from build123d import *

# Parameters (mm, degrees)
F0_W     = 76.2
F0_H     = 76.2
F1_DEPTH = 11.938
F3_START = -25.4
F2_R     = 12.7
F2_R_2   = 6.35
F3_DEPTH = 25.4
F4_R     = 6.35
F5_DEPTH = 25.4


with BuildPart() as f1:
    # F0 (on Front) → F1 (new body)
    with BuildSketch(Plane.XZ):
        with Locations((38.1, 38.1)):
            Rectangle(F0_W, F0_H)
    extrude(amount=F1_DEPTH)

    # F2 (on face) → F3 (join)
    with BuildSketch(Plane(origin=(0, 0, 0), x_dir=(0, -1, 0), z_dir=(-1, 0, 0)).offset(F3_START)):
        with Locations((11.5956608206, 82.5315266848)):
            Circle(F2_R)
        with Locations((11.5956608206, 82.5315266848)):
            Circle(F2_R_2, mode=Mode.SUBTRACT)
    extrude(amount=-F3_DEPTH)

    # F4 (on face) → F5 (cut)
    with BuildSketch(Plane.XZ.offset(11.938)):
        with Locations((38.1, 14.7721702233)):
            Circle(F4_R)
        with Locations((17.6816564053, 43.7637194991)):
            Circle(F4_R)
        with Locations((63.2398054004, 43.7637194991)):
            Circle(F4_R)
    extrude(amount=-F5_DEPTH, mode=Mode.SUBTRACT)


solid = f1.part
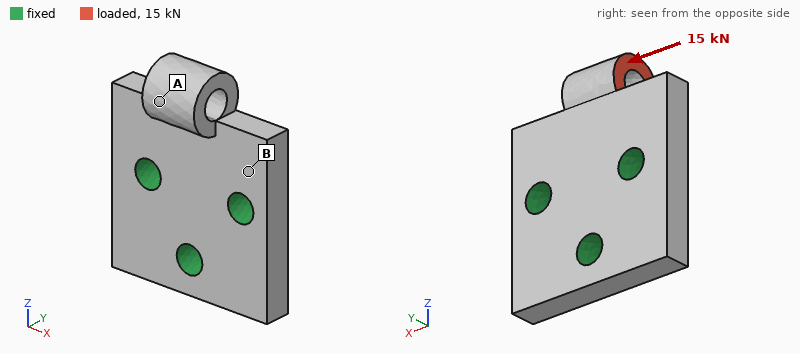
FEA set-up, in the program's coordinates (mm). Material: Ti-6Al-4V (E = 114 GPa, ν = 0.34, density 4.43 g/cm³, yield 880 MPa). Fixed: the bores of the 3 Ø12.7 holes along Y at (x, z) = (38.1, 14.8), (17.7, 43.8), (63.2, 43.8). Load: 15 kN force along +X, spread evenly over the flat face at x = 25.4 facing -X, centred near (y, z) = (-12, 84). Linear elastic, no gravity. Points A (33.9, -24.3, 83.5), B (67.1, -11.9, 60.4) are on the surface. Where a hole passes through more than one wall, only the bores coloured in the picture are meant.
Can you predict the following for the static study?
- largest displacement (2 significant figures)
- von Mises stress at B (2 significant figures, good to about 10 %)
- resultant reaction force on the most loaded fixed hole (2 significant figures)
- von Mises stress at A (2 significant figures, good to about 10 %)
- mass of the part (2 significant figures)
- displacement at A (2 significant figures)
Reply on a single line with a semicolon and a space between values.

93 µm; 26 MPa; 13 kN; 63 MPa; 320 g; 69 µm
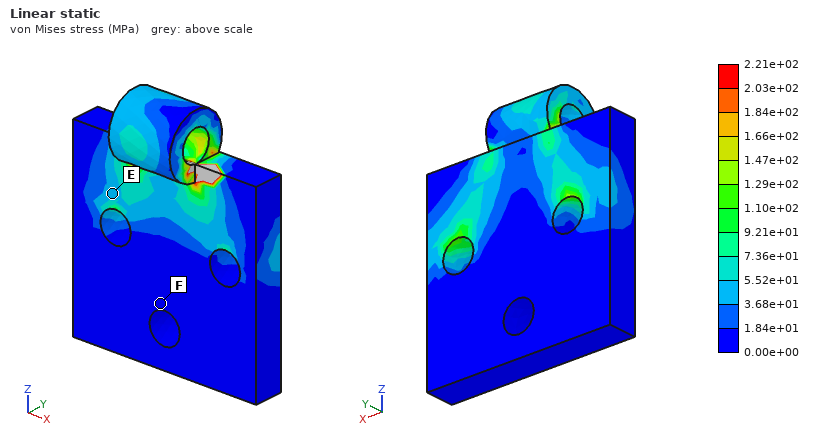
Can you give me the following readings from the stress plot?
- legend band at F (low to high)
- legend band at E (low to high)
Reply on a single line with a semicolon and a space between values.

0.00e+00 to 1.84e+01 MPa; 3.68e+01 to 5.52e+01 MPa
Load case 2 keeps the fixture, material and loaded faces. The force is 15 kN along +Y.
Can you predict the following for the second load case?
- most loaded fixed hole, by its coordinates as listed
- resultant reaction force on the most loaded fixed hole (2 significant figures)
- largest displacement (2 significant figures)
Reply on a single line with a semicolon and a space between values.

(17.7, 43.8); 14 kN; 0.55 mm
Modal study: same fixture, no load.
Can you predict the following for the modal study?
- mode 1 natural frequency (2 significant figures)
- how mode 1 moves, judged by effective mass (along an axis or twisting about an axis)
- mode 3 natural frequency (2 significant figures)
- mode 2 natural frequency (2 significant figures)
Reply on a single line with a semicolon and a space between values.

4600 Hz; along Y; 11 kHz; 11 kHz
